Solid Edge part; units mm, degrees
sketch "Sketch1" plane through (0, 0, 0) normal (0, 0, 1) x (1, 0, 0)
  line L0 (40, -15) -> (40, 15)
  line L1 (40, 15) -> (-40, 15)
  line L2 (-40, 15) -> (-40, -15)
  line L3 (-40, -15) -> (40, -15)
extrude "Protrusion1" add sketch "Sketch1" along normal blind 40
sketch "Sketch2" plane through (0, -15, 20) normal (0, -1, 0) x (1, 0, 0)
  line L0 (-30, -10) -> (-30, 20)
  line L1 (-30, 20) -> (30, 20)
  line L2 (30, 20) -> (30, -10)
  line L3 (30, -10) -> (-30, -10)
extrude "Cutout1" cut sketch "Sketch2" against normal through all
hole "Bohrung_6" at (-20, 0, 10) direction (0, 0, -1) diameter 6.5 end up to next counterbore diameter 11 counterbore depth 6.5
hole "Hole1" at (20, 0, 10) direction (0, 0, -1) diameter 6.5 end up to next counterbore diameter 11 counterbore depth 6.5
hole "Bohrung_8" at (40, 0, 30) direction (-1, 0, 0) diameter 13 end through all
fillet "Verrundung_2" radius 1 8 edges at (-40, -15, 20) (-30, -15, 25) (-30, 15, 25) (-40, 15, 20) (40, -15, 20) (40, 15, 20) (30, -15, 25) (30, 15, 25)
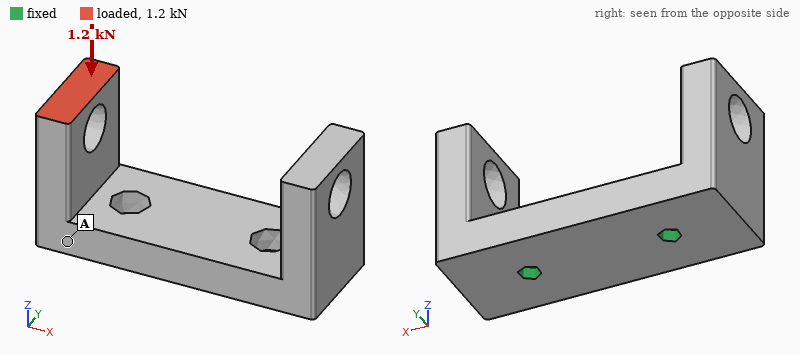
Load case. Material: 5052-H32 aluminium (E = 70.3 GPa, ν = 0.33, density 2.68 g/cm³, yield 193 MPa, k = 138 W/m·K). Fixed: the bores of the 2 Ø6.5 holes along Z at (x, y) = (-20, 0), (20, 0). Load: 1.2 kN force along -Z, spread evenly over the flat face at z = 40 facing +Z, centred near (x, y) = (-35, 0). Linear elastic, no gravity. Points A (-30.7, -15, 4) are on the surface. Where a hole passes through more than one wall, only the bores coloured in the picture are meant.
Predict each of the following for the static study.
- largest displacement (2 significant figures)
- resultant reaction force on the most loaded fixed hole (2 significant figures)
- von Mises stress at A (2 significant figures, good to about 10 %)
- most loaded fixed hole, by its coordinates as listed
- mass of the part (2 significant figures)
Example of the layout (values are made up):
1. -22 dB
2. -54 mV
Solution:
1. 71 µm
2. 1.7 kN
3. 9.2 MPa
4. (-20, 0)
5. 100 g
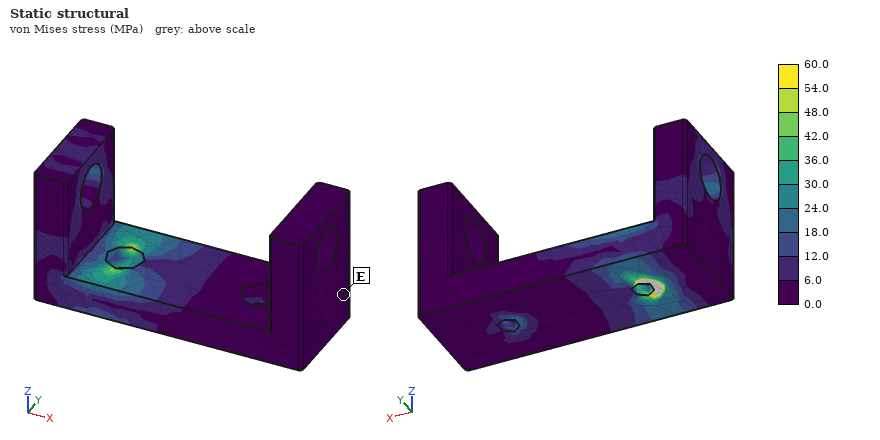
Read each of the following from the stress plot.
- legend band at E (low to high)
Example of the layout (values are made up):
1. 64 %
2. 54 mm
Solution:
1. 0.0 to 6.0 MPa
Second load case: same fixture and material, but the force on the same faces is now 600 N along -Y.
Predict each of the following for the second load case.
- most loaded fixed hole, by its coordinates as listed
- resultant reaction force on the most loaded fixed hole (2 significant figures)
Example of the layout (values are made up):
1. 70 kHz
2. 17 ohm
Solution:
1. (-20, 0)
2. 700 N
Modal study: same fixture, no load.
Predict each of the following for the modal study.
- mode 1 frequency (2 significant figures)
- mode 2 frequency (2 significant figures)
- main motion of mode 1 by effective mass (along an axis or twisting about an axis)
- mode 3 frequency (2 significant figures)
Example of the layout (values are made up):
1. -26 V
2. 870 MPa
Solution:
1. 2900 Hz
2. 3400 Hz
3. along Y
4. 3500 Hz
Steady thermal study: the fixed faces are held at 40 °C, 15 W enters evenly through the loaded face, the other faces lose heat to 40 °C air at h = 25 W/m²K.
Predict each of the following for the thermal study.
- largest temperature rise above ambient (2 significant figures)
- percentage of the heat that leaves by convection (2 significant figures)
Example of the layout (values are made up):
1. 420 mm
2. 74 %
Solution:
1. 24 K
2. 9.0 %
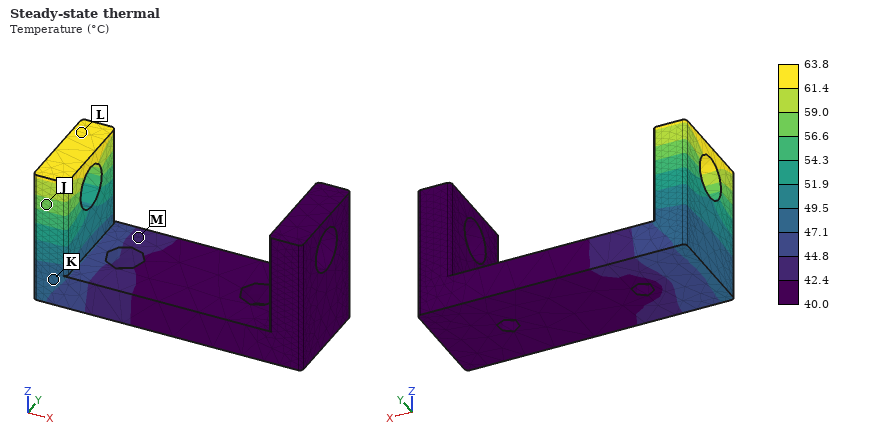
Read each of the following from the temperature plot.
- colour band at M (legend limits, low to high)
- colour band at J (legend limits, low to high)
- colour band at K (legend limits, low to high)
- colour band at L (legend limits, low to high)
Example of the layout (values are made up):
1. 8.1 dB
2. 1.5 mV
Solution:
1. 42.4 to 44.8 °C
2. 56.6 to 59.0 °C
3. 47.1 to 49.5 °C
4. 61.4 to 63.8 °C
